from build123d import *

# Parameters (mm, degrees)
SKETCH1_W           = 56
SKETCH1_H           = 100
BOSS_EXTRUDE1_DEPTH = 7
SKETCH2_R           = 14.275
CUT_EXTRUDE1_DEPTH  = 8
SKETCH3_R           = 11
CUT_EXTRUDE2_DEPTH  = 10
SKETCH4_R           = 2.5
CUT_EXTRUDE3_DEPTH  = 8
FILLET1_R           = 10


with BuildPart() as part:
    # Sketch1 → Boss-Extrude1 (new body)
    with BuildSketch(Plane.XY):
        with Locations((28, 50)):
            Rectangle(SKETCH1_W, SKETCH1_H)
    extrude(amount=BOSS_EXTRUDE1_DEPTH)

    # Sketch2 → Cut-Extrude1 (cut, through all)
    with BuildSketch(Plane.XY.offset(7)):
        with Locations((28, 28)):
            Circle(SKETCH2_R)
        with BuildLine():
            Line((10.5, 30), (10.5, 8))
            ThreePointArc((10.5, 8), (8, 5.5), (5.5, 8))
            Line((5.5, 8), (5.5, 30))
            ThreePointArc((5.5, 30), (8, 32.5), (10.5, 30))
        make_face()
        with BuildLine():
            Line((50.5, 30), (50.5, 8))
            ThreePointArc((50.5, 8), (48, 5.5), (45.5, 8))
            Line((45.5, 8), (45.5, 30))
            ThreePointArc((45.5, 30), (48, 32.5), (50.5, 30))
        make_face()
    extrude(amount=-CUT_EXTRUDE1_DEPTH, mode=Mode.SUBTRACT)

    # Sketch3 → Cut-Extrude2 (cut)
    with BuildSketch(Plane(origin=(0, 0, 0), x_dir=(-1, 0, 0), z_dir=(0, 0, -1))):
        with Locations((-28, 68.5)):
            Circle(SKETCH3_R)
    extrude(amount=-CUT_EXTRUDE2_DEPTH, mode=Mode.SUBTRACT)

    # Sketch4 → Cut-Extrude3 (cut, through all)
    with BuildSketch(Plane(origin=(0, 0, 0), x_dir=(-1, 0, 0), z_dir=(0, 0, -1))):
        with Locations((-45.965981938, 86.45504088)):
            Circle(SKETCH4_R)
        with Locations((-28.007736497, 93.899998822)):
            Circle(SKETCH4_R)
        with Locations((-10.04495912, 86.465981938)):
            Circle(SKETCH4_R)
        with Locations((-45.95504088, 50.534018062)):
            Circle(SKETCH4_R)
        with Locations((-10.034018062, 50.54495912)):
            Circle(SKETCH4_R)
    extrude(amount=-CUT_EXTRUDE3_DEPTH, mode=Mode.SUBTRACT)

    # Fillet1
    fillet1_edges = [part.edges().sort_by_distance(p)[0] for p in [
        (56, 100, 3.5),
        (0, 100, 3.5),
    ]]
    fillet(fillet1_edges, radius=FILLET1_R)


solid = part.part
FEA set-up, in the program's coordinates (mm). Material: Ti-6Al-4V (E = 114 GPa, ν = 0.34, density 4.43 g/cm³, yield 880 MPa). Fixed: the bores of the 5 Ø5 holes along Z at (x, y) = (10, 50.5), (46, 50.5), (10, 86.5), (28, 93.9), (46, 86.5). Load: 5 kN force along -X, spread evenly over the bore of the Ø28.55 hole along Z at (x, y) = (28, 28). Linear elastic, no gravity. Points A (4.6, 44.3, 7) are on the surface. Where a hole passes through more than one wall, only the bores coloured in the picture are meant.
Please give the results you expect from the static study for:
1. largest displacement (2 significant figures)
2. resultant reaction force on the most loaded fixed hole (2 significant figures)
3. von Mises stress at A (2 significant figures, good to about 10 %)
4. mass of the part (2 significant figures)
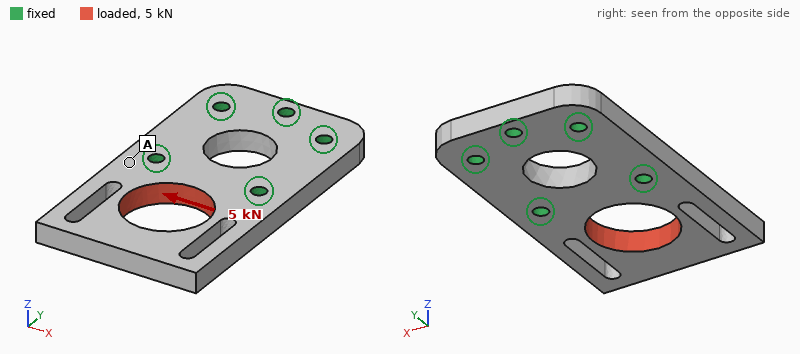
97 µm
3.3 kN
32 MPa
130 g
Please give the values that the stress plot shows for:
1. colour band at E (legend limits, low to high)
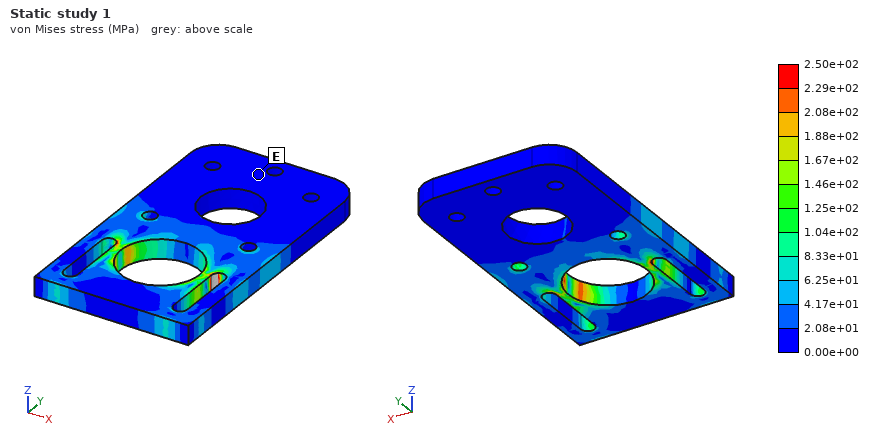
0.00e+00 to 2.08e+01 MPa
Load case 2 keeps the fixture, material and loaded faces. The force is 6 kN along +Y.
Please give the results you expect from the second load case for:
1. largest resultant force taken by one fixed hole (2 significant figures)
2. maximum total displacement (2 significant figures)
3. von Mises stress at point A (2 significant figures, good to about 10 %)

2.8 kN
15 µm
13 MPa
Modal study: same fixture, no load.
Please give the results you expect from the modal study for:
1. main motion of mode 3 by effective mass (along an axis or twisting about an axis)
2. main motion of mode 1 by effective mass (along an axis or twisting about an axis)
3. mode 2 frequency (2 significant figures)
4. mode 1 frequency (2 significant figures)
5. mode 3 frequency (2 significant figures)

along X
along Z
3900 Hz
1900 Hz
5000 Hz
